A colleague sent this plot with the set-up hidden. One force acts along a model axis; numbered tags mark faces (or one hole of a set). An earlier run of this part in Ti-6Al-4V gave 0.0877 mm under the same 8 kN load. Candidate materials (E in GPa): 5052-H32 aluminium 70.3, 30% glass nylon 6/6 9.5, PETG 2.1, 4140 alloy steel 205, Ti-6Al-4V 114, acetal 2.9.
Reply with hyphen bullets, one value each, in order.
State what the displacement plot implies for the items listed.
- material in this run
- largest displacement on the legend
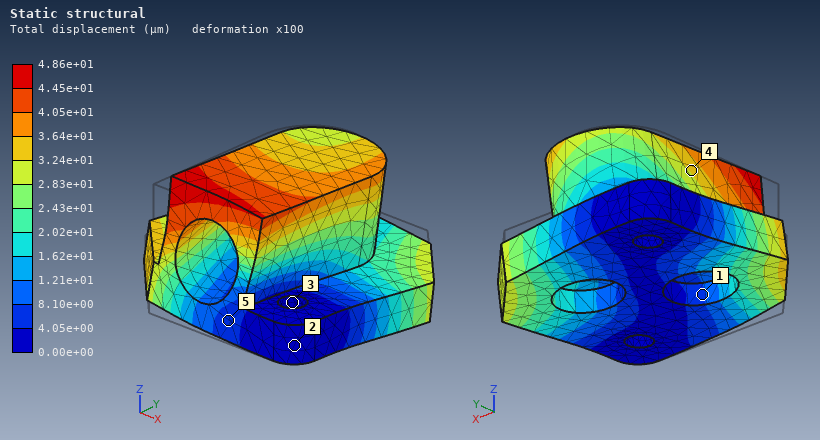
- 4140 alloy steel
- 4.86e+01 µm
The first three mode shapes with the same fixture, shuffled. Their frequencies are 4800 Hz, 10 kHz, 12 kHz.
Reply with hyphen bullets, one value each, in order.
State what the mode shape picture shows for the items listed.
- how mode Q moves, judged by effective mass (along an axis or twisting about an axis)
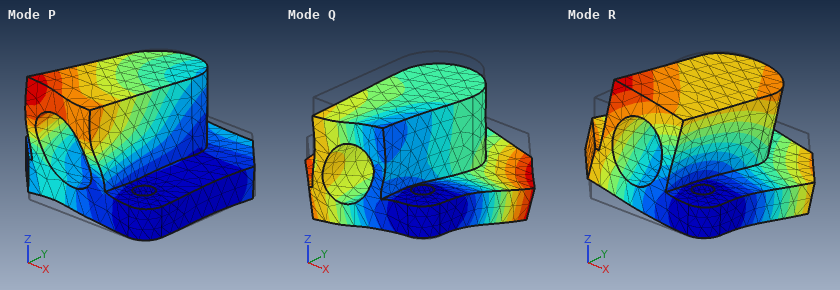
- along Z
